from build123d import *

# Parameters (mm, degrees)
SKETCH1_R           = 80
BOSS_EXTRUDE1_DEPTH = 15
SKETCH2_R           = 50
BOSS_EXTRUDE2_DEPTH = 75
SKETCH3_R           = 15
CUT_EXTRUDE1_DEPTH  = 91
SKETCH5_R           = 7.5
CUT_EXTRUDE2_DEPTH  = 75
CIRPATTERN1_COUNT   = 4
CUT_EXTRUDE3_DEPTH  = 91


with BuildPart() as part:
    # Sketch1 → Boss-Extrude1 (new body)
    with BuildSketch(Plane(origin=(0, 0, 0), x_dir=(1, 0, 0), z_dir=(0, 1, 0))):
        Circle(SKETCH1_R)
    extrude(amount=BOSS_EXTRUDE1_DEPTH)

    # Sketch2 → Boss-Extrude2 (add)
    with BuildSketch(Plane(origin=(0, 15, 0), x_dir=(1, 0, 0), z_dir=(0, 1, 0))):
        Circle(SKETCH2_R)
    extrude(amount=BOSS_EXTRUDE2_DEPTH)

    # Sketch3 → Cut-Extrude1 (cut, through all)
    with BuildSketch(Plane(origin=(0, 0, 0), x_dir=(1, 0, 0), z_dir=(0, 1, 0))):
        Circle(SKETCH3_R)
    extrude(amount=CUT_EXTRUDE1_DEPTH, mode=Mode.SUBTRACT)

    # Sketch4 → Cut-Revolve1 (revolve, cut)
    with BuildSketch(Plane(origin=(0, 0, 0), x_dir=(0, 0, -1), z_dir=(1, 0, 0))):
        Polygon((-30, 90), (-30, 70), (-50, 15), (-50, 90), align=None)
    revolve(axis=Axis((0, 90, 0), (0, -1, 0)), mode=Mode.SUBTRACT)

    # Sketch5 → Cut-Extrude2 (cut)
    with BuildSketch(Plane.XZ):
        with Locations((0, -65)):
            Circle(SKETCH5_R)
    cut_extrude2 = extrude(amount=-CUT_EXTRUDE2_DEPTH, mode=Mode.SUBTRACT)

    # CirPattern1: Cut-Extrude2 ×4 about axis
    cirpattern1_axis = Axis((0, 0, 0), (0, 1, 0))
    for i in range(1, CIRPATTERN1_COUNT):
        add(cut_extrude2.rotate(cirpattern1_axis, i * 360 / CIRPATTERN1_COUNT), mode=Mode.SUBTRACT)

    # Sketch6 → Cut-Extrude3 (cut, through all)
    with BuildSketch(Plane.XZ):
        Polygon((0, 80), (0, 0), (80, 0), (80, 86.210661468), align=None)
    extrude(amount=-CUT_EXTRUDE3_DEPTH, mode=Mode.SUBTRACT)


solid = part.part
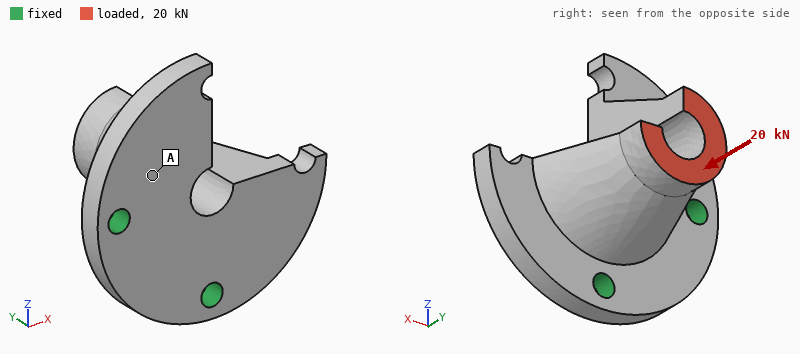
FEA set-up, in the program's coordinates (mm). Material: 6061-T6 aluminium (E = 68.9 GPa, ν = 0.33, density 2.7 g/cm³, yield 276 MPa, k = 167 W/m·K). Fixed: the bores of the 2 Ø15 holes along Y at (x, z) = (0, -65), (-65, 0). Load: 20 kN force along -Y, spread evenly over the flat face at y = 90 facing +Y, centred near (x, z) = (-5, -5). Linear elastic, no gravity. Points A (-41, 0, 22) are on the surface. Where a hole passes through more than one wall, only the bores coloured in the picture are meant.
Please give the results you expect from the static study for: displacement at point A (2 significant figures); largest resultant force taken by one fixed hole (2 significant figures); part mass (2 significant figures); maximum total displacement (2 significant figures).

0.11 mm
11 kN
1.1 kg
0.45 mm
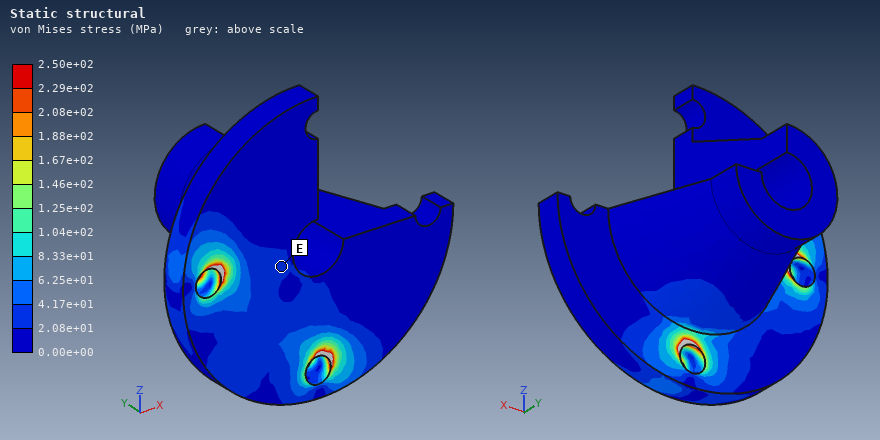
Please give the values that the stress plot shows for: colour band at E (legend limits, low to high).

2.08e+01 to 4.17e+01 MPa
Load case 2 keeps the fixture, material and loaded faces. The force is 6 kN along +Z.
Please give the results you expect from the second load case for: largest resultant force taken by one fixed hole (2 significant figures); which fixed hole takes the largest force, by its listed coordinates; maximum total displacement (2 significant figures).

6.0 kN
(0, -65)
0.26 mm
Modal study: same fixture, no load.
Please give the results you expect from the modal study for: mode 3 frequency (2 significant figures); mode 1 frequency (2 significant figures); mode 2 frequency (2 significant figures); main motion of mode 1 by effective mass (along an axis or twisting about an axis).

4200 Hz
1200 Hz
3300 Hz
along Y
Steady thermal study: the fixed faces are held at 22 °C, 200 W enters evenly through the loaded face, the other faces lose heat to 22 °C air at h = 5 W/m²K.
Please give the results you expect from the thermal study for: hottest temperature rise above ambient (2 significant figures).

56 K
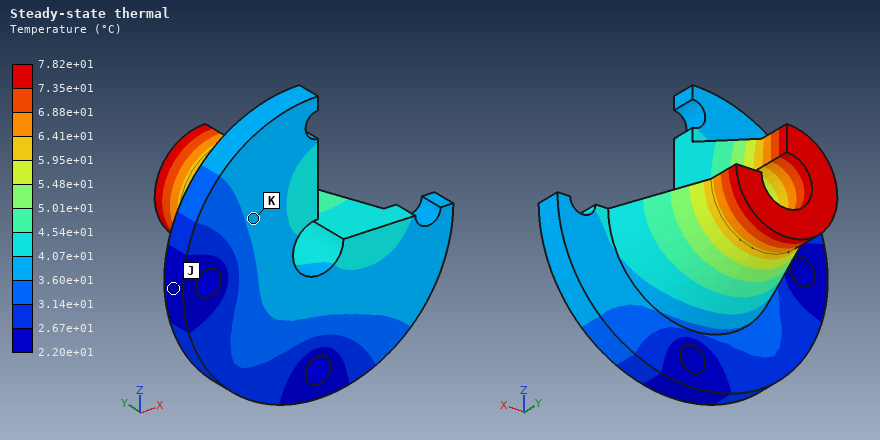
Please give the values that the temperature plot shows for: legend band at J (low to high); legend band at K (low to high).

2.20e+01 to 2.67e+01 °C
3.60e+01 to 4.07e+01 °C
